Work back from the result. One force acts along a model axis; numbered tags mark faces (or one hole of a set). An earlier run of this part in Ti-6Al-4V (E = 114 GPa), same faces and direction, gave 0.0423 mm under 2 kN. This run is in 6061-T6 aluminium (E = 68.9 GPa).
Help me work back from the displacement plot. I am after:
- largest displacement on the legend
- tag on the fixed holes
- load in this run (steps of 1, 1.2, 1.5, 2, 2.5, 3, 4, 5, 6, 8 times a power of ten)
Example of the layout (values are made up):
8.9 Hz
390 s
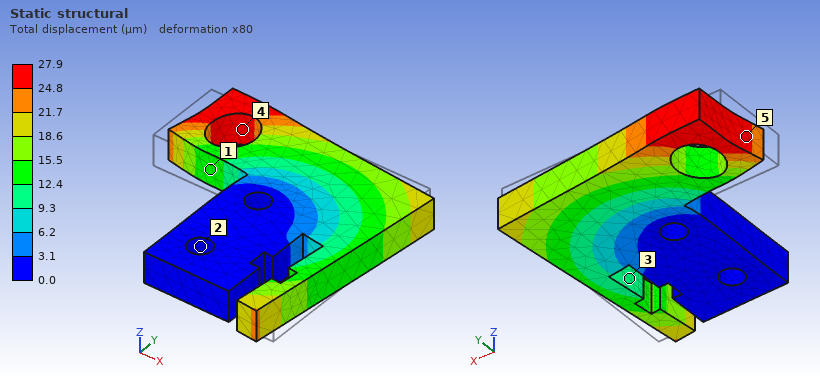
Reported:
27.9 µm
2
800 N
